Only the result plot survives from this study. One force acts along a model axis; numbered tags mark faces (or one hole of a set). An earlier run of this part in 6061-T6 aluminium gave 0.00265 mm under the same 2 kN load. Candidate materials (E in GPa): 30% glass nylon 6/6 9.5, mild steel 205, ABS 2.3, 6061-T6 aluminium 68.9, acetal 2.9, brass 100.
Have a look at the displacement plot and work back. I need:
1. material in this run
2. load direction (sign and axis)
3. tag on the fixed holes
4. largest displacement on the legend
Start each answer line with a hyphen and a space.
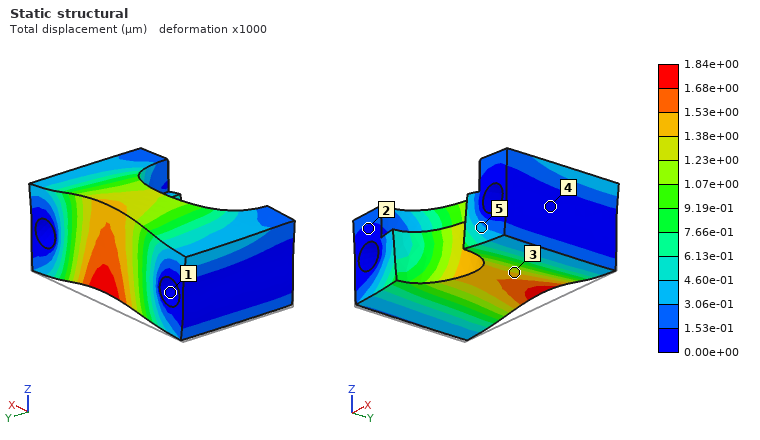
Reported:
- brass
- +Z
- 1
- 1.84e+00 µm
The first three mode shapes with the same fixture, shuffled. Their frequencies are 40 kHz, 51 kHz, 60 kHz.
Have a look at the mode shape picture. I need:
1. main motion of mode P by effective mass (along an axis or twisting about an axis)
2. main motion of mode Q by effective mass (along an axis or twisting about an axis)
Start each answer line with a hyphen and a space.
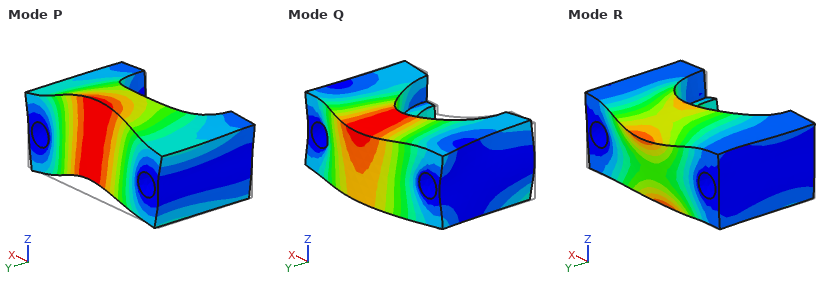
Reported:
- along Z
- along Y
